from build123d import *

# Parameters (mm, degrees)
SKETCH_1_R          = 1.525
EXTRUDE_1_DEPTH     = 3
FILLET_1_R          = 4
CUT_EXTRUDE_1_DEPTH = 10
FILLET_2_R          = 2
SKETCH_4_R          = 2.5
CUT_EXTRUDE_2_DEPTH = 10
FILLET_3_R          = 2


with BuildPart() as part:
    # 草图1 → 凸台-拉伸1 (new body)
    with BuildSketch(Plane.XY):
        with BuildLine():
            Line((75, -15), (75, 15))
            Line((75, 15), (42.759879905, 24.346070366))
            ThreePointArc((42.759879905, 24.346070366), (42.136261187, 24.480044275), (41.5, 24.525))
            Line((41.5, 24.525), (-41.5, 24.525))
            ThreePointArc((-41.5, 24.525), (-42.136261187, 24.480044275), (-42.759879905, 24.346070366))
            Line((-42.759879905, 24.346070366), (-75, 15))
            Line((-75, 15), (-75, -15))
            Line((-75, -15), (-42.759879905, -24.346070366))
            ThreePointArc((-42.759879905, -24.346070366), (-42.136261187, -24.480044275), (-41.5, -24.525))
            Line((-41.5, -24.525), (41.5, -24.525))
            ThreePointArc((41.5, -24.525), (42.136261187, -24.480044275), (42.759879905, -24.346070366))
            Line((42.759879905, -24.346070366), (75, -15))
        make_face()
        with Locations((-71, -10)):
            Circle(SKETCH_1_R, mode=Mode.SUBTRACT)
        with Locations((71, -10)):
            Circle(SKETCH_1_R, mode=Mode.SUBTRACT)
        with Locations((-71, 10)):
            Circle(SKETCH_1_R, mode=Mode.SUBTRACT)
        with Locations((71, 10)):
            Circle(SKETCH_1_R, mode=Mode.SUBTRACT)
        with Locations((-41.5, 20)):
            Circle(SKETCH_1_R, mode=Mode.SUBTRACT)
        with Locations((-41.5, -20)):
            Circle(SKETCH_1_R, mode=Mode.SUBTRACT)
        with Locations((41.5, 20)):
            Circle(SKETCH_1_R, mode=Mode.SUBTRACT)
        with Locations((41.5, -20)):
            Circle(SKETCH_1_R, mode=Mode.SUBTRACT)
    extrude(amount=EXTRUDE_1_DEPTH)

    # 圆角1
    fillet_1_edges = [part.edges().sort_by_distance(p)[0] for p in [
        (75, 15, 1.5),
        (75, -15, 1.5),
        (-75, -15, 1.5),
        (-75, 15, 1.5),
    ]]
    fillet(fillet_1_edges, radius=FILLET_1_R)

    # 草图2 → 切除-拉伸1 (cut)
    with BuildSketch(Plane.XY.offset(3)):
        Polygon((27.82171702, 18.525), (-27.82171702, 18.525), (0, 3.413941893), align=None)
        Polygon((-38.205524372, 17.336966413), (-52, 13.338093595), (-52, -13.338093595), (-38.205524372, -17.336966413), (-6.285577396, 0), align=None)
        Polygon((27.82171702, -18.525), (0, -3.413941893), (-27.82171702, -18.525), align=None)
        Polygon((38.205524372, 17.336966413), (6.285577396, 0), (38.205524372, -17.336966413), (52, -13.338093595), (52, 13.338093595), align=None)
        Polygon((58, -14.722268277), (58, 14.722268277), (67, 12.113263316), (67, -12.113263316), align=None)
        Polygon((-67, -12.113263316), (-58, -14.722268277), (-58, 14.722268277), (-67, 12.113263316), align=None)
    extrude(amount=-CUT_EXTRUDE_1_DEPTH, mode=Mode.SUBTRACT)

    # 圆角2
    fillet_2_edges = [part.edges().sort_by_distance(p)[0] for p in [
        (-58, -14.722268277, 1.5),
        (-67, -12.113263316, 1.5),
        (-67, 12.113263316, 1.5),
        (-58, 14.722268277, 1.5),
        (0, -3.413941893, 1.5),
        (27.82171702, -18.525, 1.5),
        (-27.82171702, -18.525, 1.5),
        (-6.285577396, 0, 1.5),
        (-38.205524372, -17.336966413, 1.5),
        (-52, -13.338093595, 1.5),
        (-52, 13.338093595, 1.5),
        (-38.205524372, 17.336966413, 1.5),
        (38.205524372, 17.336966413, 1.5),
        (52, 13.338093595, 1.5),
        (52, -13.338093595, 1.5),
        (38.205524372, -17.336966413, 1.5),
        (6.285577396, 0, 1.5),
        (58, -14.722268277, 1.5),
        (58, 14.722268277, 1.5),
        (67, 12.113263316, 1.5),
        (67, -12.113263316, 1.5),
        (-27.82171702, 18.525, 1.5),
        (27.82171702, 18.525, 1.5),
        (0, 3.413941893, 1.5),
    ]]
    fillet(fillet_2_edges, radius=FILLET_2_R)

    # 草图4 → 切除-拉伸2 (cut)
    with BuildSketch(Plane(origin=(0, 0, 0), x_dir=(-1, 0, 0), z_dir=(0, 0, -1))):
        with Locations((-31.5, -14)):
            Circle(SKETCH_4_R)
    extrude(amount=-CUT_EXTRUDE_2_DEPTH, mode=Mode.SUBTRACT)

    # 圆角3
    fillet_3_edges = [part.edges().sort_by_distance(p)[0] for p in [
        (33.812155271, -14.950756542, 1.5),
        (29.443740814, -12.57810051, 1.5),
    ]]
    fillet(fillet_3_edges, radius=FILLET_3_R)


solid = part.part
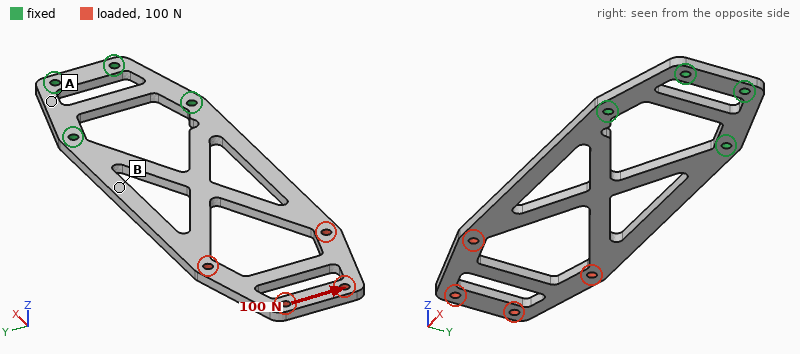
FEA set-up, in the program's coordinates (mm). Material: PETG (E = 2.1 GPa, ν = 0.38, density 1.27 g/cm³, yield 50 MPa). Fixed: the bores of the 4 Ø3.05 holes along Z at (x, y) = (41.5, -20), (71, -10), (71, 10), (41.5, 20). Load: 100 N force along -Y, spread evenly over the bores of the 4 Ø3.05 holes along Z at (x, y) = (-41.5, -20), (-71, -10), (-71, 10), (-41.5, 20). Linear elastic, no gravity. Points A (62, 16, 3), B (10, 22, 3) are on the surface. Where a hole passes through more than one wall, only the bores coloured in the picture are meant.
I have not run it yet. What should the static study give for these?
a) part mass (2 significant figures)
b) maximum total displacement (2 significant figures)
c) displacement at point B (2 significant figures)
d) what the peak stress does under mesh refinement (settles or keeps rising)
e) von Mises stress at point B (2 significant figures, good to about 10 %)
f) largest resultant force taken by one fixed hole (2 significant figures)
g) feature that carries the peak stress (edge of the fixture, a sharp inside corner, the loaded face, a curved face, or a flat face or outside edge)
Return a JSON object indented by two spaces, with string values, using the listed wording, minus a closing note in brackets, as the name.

{
  "part mass": "13 g",
  "maximum total displacement": "1.9 mm",
  "displacement at point B": "0.31 mm",
  "what the peak stress does under mesh refinement": "keeps rising",
  "von Mises stress at point B": "7.0 MPa",
  "largest resultant force taken by one fixed hole": "230 N",
  "feature that carries the peak stress": "edge of the fixture"
}
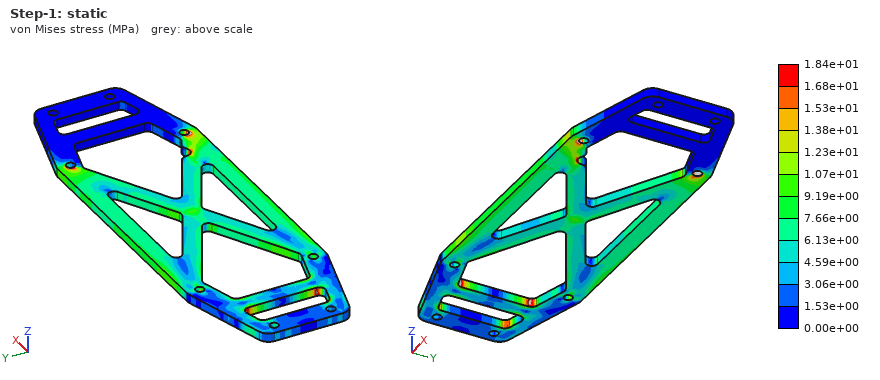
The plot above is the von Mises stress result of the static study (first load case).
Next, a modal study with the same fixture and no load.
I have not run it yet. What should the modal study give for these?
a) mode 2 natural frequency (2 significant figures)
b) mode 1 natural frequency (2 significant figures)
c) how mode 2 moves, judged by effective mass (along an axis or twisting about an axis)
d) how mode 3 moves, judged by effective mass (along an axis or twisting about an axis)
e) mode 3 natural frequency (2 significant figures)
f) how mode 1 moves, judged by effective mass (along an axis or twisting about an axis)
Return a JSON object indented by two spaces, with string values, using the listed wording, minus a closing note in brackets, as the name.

{
  "mode 2 natural frequency": "190 Hz",
  "mode 1 natural frequency": "43 Hz",
  "how mode 2 moves, judged by effective mass": "twisting about X",
  "how mode 3 moves, judged by effective mass": "along Z",
  "mode 3 natural frequency": "250 Hz",
  "how mode 1 moves, judged by effective mass": "along Z"
}
